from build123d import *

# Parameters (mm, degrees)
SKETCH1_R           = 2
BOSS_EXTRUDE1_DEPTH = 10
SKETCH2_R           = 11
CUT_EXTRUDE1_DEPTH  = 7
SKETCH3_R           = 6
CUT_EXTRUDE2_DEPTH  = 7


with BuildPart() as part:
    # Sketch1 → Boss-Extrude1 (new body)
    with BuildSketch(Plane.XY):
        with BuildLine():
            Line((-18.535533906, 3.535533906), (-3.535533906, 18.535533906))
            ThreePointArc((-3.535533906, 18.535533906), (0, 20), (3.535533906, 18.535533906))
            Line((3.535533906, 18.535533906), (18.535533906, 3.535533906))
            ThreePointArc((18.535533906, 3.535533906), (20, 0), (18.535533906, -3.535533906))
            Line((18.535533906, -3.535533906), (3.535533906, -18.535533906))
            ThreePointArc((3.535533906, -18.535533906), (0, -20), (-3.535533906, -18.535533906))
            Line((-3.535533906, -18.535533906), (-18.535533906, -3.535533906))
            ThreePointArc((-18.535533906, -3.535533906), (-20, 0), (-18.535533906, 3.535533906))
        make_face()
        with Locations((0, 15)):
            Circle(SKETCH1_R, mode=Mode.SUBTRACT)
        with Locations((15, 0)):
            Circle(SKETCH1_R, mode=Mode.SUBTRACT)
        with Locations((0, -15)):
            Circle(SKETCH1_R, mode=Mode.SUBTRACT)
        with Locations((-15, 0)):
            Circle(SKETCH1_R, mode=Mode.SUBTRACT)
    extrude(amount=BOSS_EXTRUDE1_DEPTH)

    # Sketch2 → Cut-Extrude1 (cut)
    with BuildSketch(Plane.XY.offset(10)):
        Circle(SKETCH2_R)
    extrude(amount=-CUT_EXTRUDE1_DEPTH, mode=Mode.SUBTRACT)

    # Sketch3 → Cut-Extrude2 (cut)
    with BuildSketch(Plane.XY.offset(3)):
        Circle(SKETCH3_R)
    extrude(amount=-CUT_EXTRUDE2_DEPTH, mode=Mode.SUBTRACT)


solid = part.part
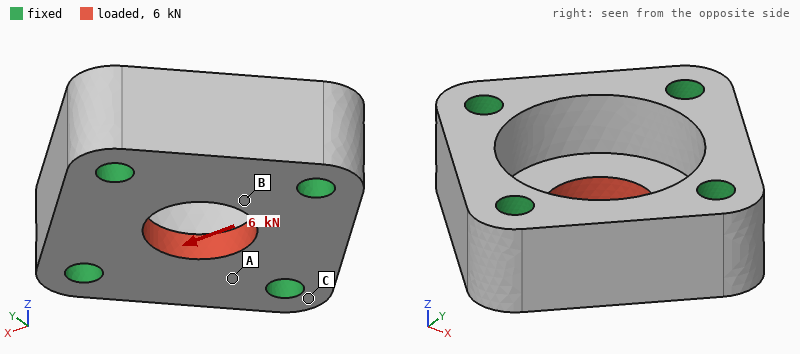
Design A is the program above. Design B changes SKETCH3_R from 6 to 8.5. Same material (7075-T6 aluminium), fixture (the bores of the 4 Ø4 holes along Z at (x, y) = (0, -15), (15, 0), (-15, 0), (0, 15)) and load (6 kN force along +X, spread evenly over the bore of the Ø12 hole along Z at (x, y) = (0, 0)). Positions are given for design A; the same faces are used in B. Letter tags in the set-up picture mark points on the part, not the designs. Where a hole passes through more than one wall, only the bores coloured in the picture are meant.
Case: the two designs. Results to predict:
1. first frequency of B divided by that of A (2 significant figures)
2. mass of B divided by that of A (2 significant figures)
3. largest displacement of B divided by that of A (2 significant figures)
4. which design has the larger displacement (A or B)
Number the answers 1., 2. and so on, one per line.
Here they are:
1. 1.0
2. 0.94
3. 0.85
4. A
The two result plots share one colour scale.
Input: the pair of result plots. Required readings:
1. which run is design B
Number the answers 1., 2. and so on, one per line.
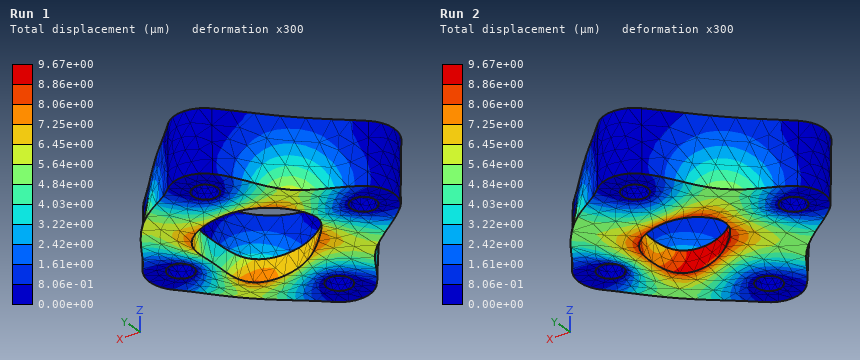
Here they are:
1. Run 1
